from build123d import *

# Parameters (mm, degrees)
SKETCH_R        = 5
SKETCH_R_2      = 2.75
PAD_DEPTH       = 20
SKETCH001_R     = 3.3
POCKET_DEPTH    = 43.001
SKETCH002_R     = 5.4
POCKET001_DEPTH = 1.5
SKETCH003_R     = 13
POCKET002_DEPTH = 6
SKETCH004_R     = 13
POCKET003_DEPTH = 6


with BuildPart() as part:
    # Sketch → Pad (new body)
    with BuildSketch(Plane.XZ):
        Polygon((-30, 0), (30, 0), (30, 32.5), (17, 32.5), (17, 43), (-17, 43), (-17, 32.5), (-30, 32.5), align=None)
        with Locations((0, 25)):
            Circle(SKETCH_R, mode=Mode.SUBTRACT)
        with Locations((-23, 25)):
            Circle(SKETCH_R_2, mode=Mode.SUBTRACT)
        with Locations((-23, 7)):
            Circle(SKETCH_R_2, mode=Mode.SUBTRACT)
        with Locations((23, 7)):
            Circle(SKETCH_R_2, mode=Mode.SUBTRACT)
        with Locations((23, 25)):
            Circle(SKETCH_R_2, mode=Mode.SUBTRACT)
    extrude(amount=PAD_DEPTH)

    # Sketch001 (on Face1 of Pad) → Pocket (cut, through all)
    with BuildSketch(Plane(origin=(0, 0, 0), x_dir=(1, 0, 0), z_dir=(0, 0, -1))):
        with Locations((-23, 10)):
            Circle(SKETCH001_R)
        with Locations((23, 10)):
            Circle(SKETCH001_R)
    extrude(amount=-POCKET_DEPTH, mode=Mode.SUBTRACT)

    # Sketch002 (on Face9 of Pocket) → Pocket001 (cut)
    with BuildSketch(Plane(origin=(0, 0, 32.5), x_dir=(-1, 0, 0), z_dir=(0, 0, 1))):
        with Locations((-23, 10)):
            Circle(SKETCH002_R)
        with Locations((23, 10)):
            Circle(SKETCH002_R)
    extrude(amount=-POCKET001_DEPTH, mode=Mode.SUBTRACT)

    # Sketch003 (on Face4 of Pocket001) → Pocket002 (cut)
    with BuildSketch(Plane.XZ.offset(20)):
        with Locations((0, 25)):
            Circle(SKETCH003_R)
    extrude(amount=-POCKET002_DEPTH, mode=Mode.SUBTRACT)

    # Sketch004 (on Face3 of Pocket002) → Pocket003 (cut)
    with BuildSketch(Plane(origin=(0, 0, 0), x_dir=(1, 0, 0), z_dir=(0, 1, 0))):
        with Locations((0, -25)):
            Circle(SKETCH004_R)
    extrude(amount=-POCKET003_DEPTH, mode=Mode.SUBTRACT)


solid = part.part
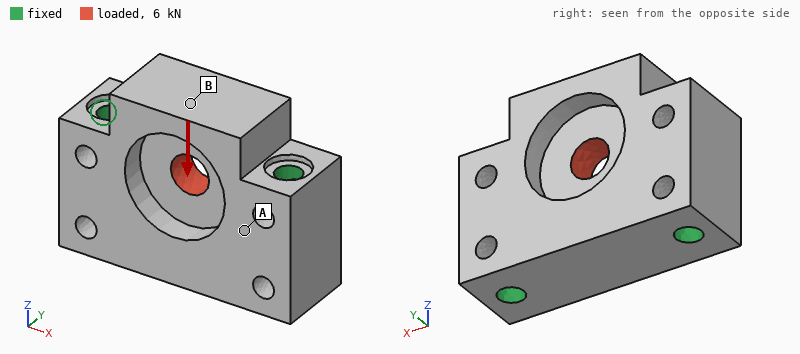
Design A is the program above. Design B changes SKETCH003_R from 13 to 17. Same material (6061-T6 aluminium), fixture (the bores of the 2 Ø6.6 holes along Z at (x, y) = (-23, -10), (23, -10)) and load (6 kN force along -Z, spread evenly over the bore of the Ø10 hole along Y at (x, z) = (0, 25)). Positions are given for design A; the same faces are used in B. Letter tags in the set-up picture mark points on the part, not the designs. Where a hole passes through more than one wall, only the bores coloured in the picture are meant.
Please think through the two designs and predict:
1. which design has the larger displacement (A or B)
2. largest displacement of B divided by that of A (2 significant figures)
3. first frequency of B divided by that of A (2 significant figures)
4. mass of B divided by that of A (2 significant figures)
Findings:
B
1.1
0.98
0.94
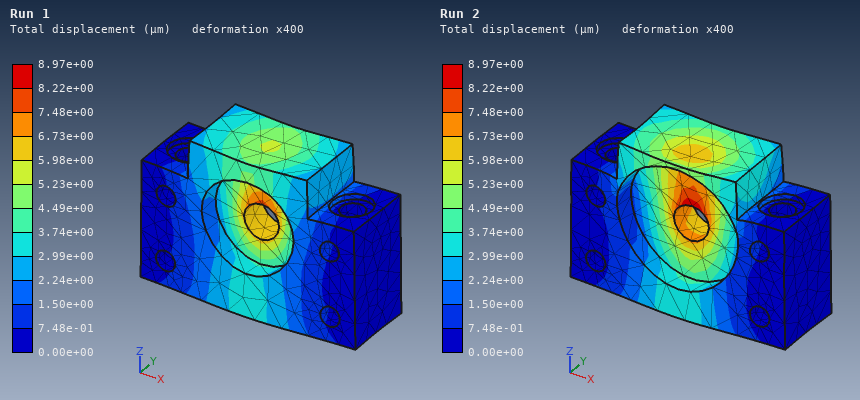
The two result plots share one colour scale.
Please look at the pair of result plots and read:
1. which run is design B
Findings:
Run 2
